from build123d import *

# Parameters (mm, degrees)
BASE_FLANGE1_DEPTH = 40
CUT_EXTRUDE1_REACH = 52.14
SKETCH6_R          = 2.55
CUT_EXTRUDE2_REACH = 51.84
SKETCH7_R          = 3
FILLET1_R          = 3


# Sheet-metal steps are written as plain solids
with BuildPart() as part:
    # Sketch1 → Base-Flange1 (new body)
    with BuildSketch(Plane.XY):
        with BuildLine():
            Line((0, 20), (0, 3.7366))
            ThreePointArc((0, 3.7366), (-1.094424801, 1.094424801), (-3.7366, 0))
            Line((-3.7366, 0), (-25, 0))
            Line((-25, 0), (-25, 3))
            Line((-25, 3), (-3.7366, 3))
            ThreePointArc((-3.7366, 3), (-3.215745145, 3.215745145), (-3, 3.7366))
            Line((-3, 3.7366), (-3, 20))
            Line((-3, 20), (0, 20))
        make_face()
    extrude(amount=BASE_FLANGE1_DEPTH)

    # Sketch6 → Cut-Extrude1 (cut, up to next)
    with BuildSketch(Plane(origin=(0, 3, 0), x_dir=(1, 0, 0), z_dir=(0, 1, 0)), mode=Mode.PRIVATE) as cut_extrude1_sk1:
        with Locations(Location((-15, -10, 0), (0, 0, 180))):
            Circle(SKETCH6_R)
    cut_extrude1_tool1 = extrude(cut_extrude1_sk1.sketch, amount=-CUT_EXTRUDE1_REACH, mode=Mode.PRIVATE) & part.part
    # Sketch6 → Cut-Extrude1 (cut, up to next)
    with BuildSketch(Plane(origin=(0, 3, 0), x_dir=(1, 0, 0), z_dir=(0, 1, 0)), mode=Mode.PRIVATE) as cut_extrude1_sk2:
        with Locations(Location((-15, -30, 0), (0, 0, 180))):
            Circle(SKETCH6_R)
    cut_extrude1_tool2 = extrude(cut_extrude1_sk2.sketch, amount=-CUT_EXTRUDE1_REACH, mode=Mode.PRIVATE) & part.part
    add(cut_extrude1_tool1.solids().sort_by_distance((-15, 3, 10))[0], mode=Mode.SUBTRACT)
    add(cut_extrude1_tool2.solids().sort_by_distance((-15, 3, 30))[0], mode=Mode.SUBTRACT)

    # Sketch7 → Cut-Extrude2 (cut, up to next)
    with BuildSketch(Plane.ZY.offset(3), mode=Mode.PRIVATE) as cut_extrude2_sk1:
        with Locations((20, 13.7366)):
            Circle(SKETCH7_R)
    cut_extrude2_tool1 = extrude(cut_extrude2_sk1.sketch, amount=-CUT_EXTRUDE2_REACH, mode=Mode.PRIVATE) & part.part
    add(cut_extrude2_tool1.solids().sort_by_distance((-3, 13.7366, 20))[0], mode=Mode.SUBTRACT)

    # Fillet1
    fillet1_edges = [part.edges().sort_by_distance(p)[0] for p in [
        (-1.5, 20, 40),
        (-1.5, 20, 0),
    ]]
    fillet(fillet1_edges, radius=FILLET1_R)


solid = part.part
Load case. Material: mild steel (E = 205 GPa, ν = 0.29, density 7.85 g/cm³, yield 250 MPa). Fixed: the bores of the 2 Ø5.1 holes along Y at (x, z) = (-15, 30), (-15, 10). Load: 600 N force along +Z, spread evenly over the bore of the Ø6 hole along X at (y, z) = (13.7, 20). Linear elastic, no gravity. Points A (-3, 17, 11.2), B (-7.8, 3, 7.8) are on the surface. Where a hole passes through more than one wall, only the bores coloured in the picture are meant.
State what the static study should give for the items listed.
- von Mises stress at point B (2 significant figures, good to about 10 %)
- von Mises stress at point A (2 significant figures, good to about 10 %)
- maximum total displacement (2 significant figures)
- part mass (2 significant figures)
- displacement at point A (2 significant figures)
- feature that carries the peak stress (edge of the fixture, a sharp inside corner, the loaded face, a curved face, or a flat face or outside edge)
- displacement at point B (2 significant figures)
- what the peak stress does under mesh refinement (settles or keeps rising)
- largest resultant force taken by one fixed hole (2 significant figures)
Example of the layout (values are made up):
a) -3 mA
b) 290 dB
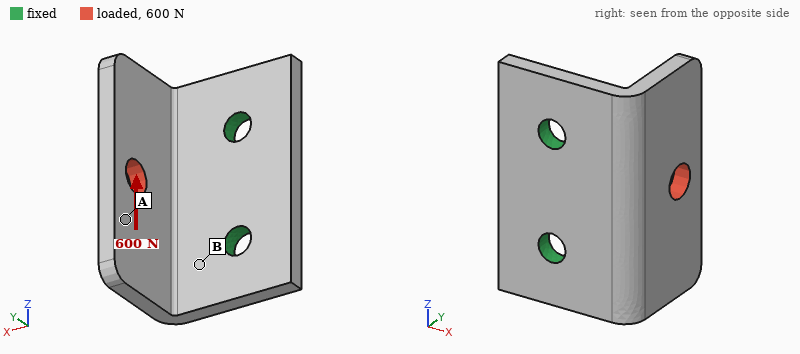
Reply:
a) 40 MPa
b) 16 MPa
c) 31 µm
d) 37 g
e) 21 µm
f) edge of the fixture
g) 5.1 µm
h) keeps rising
i) 520 N
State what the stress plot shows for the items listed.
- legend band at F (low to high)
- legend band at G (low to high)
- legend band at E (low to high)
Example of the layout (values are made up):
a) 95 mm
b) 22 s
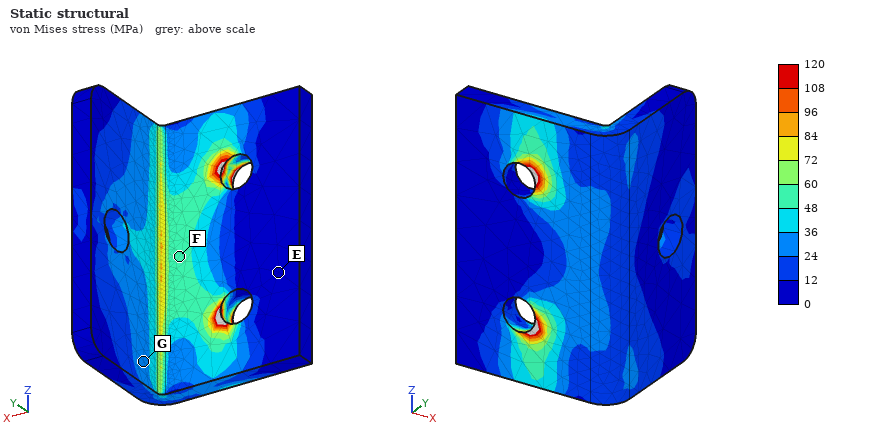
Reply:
a) 48 to 60 MPa
b) 24 to 36 MPa
c) 0 to 12 MPa
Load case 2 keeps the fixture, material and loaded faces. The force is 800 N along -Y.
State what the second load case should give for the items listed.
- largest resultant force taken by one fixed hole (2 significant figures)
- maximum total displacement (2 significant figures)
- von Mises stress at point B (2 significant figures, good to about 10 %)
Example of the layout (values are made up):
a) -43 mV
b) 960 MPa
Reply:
a) 400 N
b) 72 µm
c) 81 MPa
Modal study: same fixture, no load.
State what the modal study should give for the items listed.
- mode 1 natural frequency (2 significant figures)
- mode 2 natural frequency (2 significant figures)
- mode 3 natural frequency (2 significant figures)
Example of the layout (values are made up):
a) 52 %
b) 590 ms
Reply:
a) 3600 Hz
b) 5700 Hz
c) 9700 Hz
